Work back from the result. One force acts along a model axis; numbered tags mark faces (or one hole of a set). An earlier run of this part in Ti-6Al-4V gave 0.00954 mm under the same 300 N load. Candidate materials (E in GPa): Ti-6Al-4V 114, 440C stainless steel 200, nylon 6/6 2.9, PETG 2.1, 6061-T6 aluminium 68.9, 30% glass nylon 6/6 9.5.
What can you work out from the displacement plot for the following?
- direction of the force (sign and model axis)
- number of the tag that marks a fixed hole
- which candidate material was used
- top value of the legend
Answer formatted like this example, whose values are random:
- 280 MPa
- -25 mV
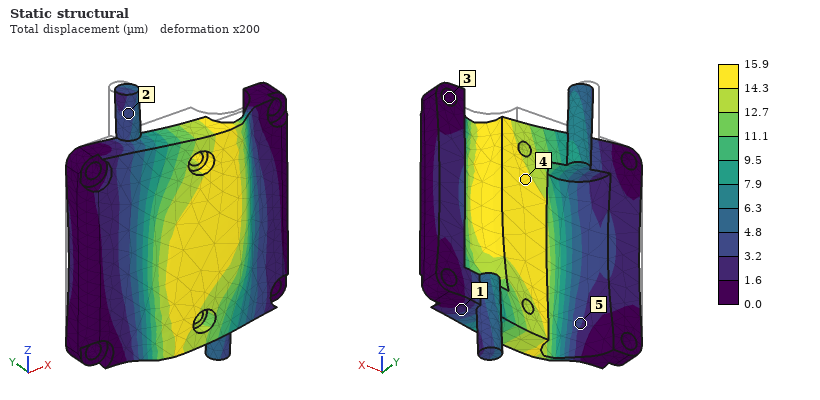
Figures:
- -Y
- 3
- 6061-T6 aluminium
- 15.9 µm
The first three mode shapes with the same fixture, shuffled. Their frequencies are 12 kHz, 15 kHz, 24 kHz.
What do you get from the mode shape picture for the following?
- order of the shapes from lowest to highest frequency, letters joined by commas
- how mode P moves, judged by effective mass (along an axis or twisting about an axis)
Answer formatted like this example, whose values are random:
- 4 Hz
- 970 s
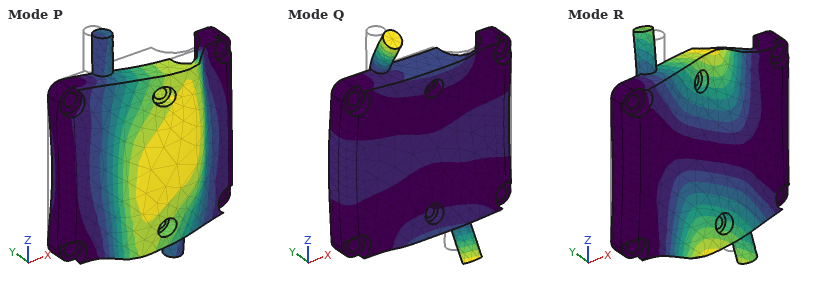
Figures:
- P, R, Q
- along Y
